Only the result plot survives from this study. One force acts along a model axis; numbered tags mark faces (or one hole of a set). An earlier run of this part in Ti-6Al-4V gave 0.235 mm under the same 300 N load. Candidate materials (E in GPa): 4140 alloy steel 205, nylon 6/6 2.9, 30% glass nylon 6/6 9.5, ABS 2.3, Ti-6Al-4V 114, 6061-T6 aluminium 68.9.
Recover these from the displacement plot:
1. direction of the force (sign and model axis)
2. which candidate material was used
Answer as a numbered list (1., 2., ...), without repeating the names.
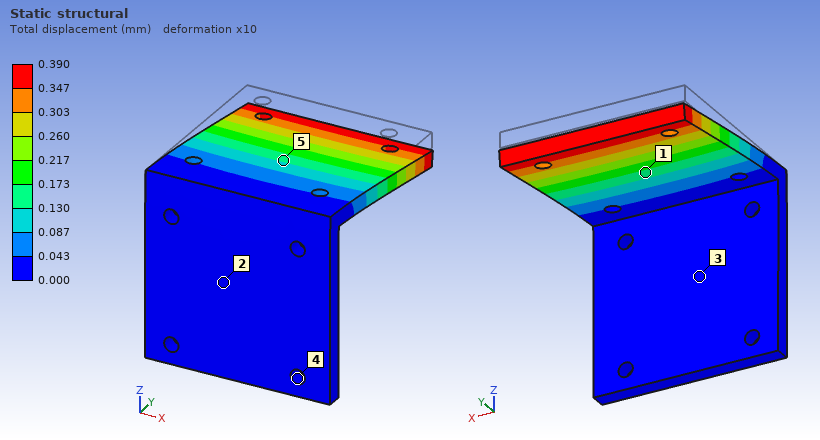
1. -Z
2. 6061-T6 aluminium
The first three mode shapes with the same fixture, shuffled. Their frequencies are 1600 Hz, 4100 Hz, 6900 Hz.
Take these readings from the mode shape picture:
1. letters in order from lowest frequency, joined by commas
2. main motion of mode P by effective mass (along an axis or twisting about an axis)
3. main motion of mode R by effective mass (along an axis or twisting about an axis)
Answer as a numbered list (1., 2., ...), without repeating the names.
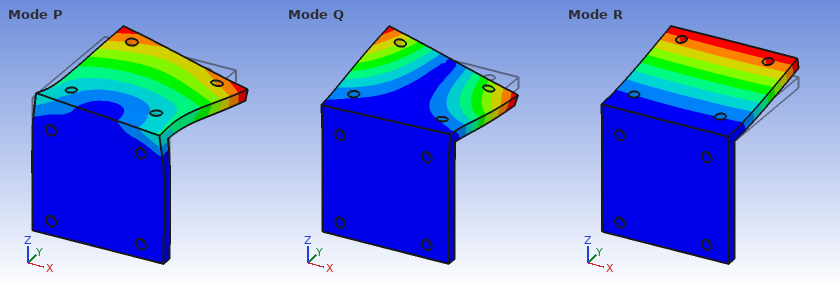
1. R, Q, P
2. along X
3. along Z
